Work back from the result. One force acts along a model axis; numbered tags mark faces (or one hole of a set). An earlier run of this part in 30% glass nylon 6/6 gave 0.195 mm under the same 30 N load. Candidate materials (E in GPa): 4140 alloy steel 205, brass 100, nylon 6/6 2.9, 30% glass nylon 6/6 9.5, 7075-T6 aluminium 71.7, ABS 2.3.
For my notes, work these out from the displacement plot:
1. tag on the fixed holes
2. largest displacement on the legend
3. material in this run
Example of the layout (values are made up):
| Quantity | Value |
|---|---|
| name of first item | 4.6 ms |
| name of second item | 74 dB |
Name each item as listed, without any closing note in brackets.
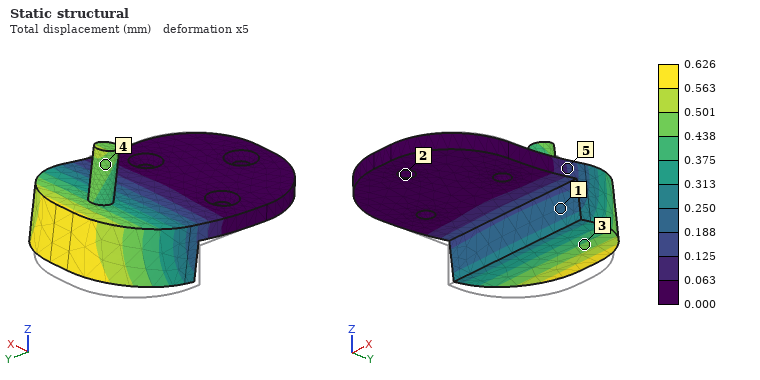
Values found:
| Quantity | Value |
|---|---|
| tag on the fixed holes | 2 |
| largest displacement on the legend | 0.626 mm |
| material in this run | nylon 6/6 |
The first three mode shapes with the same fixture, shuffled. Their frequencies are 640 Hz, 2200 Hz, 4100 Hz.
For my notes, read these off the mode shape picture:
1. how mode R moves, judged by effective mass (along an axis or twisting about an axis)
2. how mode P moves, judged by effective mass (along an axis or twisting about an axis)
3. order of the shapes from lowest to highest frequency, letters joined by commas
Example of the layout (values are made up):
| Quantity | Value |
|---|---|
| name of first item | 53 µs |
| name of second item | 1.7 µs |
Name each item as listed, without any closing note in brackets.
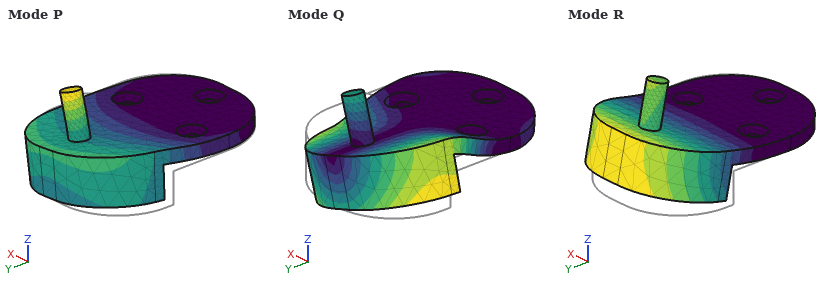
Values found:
| Quantity | Value |
|---|---|
| how mode R moves, judged by effective mass | along Z |
| how mode P moves, judged by effective mass | along X |
| order of the shapes from lowest to highest frequency, letters joined by commas | R, Q, P |
